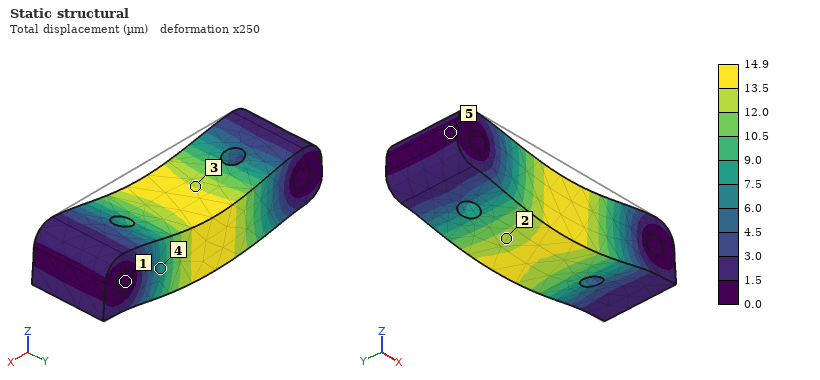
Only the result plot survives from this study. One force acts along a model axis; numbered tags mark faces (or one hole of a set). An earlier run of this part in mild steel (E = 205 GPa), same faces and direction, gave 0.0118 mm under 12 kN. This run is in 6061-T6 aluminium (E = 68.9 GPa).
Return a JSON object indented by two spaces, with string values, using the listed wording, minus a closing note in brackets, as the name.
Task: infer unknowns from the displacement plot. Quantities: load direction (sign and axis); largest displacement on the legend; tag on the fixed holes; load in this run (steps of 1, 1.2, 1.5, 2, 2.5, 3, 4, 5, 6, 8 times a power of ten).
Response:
{
  "load direction": "-Z",
  "largest displacement on the legend": "14.9 µm",
  "tag on the fixed holes": "1",
  "load in this run": "5 kN"
}
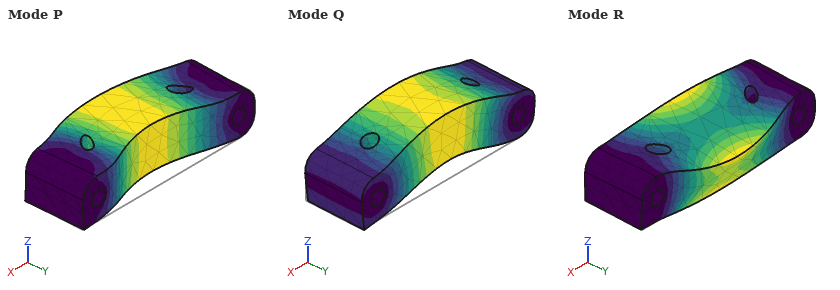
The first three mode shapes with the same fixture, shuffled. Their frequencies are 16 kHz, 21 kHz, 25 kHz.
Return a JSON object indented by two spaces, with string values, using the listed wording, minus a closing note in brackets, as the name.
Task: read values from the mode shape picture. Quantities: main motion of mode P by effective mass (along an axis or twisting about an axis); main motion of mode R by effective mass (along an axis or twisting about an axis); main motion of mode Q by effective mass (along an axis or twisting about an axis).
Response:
{
  "main motion of mode P by effective mass": "along Y",
  "main motion of mode R by effective mass": "twisting about X",
  "main motion of mode Q by effective mass": "along Z"
}
